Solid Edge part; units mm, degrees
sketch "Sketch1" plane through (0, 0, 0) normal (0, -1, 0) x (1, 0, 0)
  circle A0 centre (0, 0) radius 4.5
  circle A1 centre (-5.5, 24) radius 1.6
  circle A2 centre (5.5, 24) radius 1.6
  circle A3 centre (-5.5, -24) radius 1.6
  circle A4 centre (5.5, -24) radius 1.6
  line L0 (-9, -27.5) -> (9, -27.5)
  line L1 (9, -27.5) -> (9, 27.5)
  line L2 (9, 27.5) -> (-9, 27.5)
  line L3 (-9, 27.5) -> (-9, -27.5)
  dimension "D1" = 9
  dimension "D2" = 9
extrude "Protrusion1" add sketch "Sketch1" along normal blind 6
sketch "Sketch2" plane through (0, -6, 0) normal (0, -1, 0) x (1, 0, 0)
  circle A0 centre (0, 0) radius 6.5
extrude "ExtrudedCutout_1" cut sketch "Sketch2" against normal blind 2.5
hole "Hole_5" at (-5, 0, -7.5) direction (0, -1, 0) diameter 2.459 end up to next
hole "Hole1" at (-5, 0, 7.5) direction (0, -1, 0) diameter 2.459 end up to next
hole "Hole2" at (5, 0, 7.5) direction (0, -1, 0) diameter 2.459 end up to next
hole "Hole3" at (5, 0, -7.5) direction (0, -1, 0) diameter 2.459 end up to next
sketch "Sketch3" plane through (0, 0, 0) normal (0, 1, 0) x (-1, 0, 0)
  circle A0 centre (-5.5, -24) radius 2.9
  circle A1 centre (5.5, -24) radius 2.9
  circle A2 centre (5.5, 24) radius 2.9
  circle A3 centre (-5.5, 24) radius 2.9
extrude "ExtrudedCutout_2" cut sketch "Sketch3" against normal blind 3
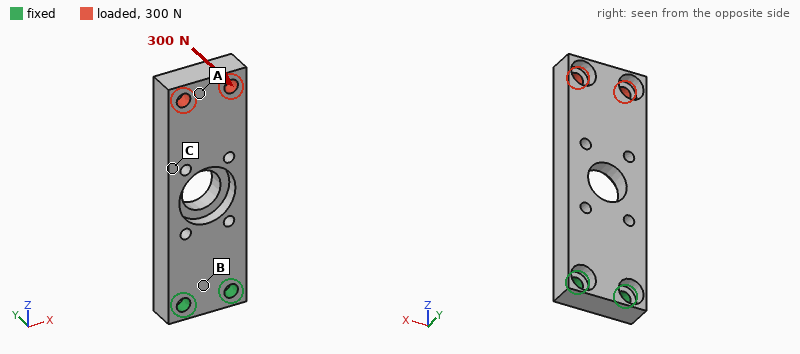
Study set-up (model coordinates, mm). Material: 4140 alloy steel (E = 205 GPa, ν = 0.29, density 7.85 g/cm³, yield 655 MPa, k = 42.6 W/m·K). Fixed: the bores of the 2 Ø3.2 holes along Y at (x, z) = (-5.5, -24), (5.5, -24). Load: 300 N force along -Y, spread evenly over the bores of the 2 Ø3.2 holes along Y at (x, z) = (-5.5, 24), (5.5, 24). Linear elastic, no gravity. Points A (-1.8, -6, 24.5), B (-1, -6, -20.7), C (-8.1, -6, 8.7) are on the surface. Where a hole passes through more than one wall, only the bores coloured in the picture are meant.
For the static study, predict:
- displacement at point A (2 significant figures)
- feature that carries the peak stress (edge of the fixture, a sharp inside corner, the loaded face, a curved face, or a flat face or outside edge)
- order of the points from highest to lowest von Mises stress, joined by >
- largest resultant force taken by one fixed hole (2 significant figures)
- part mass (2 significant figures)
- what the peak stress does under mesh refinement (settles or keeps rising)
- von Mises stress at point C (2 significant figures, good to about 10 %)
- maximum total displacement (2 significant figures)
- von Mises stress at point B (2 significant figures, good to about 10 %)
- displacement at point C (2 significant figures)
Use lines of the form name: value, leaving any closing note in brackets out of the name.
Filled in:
displacement at point A: 0.32 mm
feature that carries the peak stress: edge of the fixture
order of the points from highest to lowest von Mises stress, joined by >: B > C > A
largest resultant force taken by one fixed hole: 170 N
part mass: 38 g
what the peak stress does under mesh refinement: keeps rising
von Mises stress at point C: 79 MPa
maximum total displacement: 0.35 mm
von Mises stress at point B: 140 MPa
displacement at point C: 0.17 mm
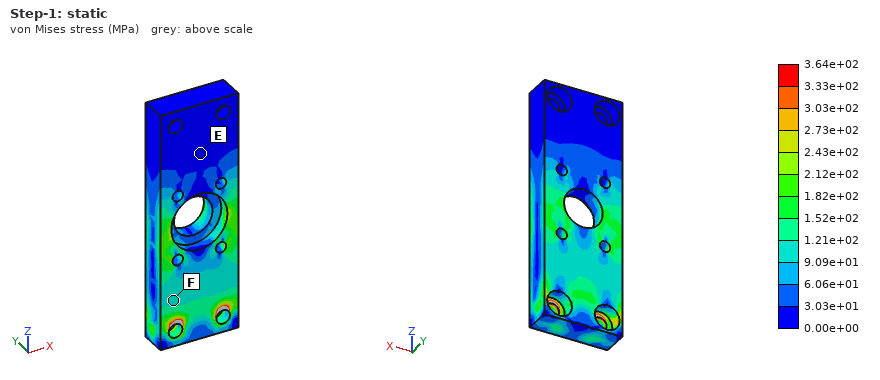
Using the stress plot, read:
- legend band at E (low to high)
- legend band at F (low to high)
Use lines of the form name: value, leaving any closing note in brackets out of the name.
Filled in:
legend band at E: 0.00e+00 to 3.03e+01 MPa
legend band at F: 9.09e+01 to 1.21e+02 MPa
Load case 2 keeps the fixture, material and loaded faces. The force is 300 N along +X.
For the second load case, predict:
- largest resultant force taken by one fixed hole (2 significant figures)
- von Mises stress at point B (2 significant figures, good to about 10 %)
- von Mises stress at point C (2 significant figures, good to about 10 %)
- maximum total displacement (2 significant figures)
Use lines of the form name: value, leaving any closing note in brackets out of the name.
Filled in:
largest resultant force taken by one fixed hole: 1.1 kN
von Mises stress at point B: 25 MPa
von Mises stress at point C: 17 MPa
maximum total displacement: 36 µm
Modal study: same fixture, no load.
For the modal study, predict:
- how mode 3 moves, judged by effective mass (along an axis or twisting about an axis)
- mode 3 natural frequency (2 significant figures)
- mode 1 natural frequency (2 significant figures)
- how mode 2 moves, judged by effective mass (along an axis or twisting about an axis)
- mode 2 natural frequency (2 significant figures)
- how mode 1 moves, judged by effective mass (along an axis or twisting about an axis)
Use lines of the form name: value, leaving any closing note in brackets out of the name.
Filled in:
how mode 3 moves, judged by effective mass: twisting about Z
mode 3 natural frequency: 7800 Hz
mode 1 natural frequency: 1500 Hz
how mode 2 moves, judged by effective mass: along X
mode 2 natural frequency: 4600 Hz
how mode 1 moves, judged by effective mass: along Y
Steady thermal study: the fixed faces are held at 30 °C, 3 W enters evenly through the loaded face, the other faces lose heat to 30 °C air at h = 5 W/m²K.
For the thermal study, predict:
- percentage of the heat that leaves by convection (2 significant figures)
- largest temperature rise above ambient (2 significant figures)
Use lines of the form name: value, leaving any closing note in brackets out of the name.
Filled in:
percentage of the heat that leaves by convection: 11 %
largest temperature rise above ambient: 43 K
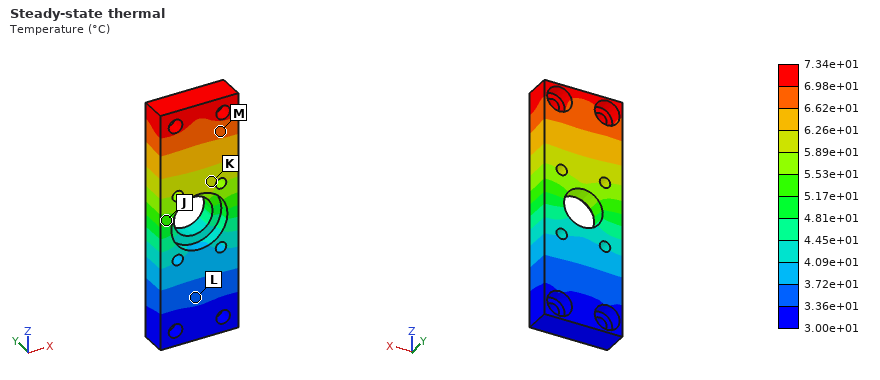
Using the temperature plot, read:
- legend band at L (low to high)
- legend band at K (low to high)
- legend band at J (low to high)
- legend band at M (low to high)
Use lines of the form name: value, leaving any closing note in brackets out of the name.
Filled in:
legend band at L: 3.36e+01 to 3.72e+01 °C
legend band at K: 5.89e+01 to 6.26e+01 °C
legend band at J: 5.17e+01 to 5.53e+01 °C
legend band at M: 6.62e+01 to 6.98e+01 °C
